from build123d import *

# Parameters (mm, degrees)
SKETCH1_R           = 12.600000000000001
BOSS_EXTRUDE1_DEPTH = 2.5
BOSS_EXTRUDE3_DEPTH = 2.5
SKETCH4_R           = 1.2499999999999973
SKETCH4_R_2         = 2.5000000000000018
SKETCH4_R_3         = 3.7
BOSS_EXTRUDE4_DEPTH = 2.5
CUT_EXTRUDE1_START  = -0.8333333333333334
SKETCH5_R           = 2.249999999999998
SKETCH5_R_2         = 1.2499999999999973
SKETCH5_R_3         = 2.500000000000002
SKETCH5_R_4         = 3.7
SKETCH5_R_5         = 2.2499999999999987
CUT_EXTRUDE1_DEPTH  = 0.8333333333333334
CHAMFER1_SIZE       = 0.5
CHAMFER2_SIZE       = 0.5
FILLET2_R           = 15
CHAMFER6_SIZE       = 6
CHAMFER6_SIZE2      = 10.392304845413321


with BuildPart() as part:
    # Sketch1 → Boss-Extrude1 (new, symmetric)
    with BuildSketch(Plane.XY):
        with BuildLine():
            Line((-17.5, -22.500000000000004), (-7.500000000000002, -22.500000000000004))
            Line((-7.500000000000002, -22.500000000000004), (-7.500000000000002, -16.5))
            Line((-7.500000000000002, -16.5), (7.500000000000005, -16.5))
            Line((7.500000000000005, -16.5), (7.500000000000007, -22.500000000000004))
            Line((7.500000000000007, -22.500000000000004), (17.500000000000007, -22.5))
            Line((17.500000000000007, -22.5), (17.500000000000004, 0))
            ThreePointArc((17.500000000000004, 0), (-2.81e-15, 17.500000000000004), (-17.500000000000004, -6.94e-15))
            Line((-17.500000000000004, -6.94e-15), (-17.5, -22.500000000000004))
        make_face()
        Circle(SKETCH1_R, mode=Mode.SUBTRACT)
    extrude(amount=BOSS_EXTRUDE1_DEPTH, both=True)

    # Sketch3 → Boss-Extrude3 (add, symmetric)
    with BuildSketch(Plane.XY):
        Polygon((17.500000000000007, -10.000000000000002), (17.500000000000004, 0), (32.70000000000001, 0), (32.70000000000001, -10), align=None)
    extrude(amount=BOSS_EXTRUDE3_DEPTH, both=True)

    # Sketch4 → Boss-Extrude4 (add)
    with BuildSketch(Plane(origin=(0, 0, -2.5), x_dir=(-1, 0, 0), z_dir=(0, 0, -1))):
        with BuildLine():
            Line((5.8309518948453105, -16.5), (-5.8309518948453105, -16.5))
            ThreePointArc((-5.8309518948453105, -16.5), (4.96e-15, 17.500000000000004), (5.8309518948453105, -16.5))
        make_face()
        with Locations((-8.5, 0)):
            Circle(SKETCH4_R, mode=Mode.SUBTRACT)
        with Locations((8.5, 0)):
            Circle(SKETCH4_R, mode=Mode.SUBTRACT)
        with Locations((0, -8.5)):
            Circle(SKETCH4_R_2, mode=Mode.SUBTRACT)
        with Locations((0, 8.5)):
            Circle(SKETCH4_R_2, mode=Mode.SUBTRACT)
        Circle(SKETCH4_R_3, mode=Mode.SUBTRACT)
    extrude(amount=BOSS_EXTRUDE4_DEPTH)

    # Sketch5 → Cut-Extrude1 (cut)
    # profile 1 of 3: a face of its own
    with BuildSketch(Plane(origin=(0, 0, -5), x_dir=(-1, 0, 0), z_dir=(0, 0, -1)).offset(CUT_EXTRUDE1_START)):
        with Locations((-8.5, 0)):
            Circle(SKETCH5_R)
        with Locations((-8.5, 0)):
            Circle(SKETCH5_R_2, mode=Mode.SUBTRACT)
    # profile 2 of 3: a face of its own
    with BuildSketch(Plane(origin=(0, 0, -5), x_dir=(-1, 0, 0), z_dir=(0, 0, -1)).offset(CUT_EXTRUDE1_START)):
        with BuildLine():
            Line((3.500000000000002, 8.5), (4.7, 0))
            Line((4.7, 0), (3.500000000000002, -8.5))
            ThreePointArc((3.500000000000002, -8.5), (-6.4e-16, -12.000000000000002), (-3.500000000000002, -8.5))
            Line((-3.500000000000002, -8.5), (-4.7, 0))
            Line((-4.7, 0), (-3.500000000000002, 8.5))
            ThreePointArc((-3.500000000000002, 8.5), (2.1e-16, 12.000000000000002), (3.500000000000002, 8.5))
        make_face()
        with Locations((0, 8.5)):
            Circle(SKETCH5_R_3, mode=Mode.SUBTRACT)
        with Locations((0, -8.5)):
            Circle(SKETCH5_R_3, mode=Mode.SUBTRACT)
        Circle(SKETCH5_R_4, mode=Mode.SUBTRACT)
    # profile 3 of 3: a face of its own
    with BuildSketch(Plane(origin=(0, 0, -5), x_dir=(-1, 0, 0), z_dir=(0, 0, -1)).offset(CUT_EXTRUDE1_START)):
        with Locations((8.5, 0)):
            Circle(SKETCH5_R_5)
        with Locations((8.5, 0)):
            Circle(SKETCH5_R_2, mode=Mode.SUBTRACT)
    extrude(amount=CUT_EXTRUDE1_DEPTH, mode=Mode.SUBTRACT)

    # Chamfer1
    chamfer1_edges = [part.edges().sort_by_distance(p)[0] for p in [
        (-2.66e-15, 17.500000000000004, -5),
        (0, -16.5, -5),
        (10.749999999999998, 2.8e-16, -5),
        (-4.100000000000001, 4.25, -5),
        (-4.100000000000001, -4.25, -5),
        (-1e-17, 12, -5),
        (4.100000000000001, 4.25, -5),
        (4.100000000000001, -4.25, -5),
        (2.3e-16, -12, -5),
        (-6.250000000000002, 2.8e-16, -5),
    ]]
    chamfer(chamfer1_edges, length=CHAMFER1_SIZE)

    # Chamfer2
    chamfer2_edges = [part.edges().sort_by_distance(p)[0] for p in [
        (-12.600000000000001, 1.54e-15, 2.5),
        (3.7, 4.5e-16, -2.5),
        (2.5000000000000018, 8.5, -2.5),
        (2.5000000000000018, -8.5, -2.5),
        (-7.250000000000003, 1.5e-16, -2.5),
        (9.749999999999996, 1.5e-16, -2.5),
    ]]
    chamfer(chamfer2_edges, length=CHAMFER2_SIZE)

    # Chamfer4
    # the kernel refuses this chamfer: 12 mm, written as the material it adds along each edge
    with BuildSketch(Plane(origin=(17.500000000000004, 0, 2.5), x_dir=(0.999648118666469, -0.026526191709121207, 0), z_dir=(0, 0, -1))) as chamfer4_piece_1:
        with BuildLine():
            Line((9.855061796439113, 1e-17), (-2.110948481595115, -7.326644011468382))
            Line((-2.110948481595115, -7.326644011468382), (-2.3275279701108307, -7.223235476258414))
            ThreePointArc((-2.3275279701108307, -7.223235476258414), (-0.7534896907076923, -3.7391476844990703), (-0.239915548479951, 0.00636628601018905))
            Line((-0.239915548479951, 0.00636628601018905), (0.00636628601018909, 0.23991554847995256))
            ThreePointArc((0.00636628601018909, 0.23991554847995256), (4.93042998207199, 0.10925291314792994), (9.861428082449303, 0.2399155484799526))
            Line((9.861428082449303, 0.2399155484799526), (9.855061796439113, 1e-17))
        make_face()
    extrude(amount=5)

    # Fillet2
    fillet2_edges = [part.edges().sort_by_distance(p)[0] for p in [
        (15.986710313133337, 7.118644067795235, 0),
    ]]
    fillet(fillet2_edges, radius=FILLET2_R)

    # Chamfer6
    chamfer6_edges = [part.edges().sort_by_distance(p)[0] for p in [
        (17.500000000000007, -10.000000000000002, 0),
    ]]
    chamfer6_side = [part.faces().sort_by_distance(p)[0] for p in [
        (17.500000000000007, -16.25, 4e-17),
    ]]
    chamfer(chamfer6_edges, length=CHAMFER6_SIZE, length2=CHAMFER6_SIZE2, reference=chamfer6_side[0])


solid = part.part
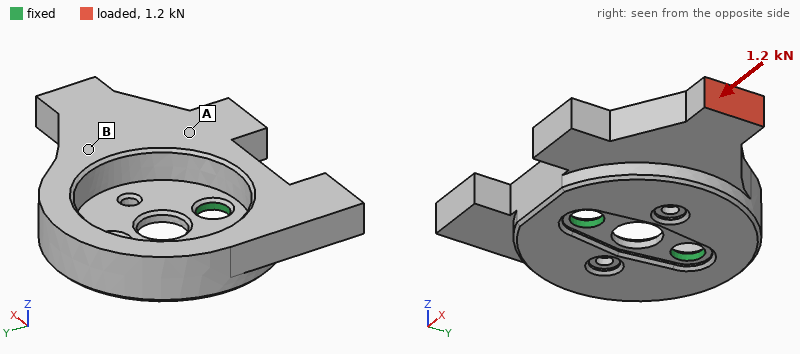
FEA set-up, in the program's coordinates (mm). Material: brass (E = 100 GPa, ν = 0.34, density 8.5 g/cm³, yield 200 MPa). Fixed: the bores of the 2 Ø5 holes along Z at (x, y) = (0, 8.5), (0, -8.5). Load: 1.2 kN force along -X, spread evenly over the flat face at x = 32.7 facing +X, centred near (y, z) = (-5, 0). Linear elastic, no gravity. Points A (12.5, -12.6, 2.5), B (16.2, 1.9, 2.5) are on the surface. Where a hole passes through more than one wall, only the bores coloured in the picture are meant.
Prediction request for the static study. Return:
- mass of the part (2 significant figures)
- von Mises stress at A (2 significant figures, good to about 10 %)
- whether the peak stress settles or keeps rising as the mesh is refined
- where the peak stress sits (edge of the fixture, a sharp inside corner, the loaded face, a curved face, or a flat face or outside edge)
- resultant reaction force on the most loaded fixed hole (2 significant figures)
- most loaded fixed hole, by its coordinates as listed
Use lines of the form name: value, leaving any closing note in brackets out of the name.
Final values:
mass of the part: 55 g
von Mises stress at A: 28 MPa
whether the peak stress settles or keeps rising as the mesh is refined: keeps rising
where the peak stress sits: edge of the fixture
resultant reaction force on the most loaded fixed hole: 920 N
most loaded fixed hole, by its coordinates as listed: (0, -8.5)
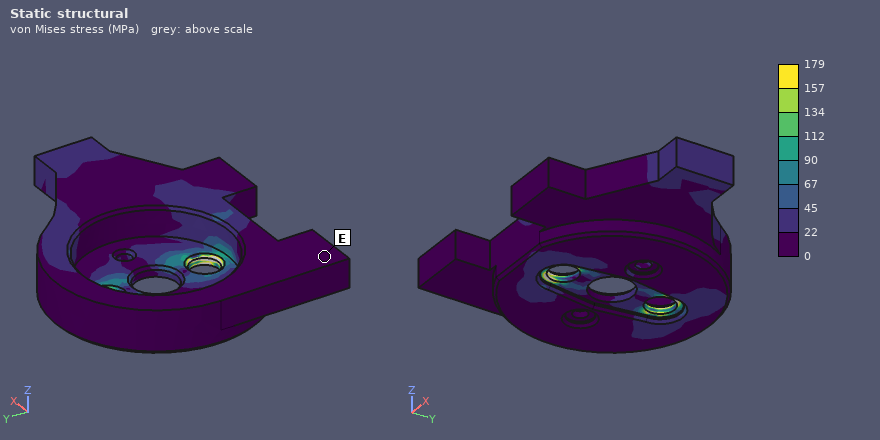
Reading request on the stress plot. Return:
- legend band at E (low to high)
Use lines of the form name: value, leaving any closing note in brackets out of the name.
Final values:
legend band at E: 0 to 22 MPa
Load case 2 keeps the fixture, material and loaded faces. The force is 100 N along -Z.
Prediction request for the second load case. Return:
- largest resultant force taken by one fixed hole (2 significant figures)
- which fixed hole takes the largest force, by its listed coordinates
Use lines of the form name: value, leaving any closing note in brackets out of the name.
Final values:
largest resultant force taken by one fixed hole: 76 N
which fixed hole takes the largest force, by its listed coordinates: (0, -8.5)
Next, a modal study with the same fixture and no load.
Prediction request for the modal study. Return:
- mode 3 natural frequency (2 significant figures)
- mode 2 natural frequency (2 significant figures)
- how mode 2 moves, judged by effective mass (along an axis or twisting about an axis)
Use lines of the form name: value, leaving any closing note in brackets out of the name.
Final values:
mode 3 natural frequency: 6800 Hz
mode 2 natural frequency: 5200 Hz
how mode 2 moves, judged by effective mass: along Z
